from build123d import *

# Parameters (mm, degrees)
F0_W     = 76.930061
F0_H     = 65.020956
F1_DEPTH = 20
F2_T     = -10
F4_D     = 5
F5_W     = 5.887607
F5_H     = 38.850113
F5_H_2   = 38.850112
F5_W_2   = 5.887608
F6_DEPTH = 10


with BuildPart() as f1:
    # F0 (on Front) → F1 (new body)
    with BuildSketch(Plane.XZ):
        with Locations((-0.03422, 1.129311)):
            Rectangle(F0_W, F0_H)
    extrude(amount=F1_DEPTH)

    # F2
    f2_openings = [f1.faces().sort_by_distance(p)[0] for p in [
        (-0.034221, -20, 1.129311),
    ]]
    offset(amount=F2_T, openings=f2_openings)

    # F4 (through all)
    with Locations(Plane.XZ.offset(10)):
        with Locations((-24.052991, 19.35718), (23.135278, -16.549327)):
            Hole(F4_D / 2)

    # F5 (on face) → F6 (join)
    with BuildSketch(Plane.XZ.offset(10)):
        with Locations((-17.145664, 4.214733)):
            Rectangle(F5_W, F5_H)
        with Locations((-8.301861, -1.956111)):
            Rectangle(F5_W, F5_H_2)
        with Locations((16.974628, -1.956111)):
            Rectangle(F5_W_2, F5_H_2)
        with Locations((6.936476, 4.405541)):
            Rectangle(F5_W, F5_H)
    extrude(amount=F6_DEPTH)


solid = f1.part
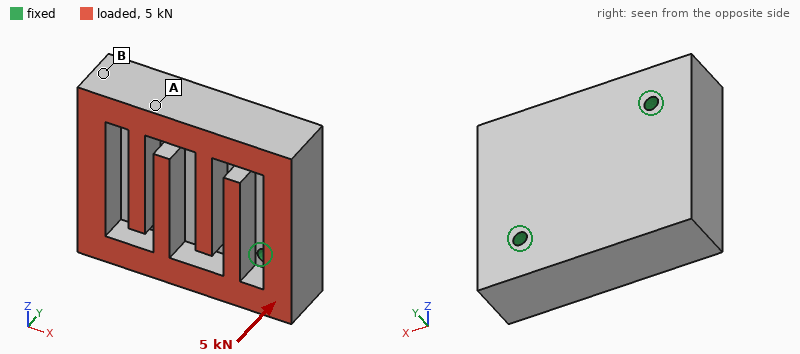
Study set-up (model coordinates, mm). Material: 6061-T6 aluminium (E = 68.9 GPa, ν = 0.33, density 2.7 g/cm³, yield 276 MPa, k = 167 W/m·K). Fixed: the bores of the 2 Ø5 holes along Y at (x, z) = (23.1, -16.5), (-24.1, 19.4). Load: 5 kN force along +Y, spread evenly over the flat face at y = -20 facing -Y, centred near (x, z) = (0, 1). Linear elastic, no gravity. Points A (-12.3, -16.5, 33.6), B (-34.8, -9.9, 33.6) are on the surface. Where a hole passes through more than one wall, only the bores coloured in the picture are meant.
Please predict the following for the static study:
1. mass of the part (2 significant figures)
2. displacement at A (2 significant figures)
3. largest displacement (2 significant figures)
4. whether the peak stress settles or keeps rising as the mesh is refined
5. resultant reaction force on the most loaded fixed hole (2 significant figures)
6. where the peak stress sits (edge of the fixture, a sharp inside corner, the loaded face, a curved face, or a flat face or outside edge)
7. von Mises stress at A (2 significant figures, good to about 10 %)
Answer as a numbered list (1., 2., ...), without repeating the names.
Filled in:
1. 220 g
2. 6.7 µm
3. 38 µm
4. keeps rising
5. 2.5 kN
6. edge of the fixture
7. 9.5 MPa
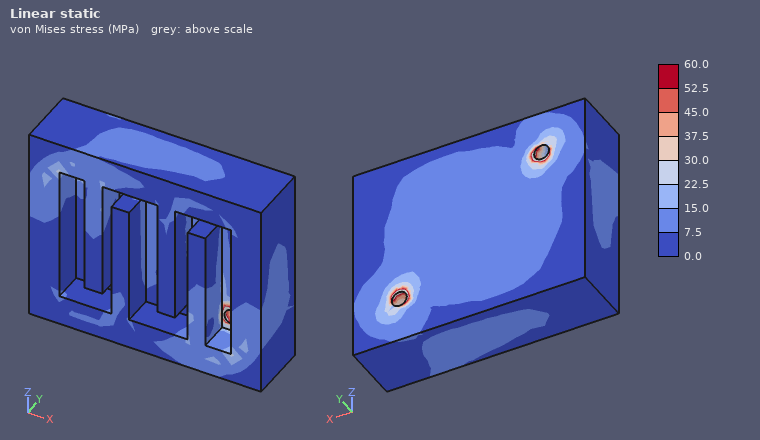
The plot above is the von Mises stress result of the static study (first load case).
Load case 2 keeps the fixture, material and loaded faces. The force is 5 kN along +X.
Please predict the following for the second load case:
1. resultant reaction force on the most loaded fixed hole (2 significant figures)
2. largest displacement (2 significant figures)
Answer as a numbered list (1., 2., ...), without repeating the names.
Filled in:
1. 2.7 kN
2. 50 µm
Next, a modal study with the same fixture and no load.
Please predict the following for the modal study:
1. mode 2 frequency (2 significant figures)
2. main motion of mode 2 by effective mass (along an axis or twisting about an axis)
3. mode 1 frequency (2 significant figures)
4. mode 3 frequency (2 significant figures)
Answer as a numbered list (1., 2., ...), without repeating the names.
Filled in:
1. 5200 Hz
2. along Y
3. 3500 Hz
4. 12 kHz
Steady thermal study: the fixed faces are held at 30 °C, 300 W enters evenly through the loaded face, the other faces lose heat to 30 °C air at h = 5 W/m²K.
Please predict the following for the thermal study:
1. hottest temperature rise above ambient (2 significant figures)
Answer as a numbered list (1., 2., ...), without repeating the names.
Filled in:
1. 44 K
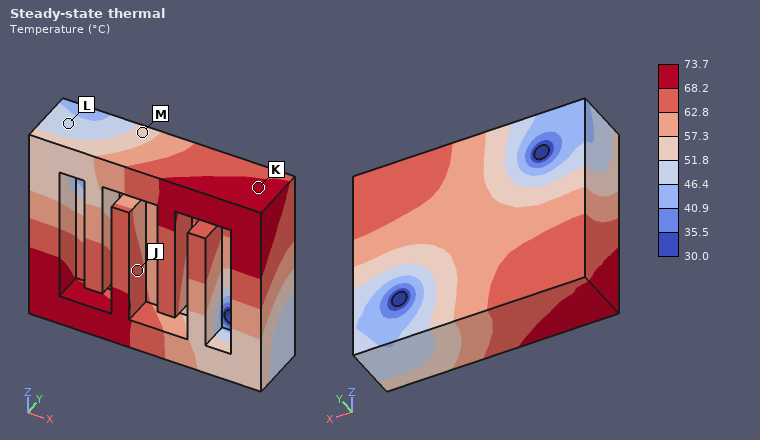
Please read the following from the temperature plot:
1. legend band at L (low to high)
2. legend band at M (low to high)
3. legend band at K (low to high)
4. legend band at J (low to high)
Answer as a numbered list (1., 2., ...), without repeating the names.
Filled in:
1. 46.4 to 51.8 °C
2. 51.8 to 57.3 °C
3. 68.2 to 73.7 °C
4. 62.8 to 68.2 °C
